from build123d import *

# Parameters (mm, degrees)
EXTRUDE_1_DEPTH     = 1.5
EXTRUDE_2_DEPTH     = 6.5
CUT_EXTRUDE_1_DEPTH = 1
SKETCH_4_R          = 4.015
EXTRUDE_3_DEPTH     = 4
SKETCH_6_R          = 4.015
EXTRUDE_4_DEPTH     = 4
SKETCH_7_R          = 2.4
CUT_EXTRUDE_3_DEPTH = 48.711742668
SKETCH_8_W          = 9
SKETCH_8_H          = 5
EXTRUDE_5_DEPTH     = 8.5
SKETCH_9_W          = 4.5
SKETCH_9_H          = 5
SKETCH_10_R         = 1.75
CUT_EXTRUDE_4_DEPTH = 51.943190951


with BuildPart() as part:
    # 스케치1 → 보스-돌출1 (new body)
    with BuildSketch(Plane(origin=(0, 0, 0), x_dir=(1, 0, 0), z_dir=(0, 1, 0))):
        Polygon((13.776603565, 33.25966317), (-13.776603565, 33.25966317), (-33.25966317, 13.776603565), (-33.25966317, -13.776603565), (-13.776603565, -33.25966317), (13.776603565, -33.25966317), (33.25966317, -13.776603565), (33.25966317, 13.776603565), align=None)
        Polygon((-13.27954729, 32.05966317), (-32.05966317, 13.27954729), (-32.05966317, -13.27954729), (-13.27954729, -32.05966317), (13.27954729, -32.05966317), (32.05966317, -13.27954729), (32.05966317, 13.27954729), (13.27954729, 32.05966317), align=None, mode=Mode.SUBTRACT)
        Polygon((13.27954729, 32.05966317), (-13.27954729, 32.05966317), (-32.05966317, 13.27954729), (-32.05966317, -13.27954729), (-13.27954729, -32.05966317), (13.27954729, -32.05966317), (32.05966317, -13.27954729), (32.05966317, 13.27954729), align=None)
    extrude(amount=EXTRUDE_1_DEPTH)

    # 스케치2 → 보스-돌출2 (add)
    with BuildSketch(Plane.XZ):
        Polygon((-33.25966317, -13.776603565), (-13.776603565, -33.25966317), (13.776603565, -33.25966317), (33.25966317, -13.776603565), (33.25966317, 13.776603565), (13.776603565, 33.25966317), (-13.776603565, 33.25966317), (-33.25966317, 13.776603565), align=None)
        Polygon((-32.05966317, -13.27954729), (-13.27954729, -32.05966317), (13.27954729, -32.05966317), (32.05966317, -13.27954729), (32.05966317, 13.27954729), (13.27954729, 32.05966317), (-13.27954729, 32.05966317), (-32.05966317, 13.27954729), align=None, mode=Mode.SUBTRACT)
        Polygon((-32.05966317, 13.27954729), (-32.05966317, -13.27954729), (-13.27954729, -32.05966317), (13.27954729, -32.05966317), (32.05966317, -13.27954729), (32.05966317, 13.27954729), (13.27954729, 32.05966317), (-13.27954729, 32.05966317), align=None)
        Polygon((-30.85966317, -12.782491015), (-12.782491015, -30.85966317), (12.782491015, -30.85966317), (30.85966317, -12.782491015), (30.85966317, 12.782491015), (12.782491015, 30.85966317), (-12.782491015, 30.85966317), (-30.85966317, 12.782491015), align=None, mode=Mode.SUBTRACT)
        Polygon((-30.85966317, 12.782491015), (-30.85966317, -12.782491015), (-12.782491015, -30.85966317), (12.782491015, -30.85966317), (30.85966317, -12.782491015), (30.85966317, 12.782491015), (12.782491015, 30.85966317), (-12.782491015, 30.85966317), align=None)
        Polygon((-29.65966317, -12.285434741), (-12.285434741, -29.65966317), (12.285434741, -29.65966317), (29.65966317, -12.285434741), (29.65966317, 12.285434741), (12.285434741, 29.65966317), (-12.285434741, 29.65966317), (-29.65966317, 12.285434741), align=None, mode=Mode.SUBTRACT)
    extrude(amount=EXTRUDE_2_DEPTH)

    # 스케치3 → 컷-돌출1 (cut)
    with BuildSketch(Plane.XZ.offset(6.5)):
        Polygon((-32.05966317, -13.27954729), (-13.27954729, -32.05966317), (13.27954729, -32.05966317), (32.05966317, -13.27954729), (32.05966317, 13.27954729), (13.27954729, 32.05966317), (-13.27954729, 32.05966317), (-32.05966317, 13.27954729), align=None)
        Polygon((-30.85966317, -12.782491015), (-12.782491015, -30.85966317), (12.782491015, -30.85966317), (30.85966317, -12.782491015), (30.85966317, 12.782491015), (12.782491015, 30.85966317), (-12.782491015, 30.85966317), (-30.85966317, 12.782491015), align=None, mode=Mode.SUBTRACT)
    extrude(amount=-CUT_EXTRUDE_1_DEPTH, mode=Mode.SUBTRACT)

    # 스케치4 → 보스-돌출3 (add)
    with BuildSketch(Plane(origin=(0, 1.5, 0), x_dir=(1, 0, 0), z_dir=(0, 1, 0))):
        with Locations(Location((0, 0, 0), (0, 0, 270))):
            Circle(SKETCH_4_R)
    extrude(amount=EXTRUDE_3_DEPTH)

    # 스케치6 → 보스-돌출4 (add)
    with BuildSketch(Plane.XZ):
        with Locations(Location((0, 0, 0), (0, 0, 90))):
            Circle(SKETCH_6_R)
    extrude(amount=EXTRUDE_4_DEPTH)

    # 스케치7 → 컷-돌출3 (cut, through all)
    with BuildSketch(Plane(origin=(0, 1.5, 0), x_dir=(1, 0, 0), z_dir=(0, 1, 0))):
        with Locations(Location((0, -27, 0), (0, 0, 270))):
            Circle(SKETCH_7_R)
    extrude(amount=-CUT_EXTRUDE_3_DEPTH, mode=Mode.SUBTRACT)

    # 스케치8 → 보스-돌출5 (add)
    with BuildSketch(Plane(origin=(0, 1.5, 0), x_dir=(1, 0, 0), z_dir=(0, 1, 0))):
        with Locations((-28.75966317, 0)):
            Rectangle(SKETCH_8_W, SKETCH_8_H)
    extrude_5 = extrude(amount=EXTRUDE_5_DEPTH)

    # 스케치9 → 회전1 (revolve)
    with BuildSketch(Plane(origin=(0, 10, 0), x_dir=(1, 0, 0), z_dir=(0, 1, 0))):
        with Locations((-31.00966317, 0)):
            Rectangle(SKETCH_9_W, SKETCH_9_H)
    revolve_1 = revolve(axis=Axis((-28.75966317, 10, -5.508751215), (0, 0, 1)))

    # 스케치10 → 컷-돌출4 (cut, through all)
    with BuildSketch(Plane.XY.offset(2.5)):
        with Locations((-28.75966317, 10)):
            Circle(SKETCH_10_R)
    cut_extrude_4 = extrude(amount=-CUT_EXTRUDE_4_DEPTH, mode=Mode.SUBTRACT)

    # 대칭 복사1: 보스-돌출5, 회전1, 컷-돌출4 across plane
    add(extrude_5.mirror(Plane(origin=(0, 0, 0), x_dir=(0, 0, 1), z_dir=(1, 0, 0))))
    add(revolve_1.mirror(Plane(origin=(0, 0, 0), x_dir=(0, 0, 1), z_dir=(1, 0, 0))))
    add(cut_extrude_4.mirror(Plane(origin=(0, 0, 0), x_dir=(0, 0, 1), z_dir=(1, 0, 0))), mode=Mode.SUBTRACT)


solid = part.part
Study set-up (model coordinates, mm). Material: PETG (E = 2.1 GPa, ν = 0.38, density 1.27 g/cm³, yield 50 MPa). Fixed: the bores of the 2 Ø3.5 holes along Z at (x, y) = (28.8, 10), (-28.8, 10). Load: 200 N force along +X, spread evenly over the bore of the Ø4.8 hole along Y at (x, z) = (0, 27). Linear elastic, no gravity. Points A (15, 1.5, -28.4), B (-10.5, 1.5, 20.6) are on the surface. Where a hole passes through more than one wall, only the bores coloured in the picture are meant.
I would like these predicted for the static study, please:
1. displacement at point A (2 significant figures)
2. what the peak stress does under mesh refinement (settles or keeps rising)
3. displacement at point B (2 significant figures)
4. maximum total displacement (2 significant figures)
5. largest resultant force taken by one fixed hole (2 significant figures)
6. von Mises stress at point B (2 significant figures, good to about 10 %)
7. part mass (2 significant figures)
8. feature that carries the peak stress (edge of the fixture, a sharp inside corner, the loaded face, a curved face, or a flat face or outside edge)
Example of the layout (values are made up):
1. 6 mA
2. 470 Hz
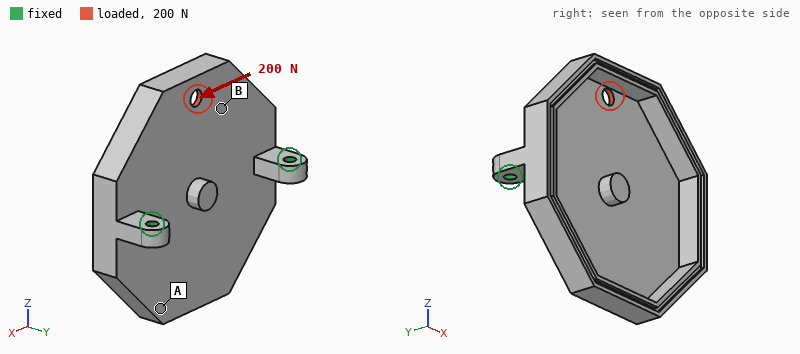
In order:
1. 0.13 mm
2. keeps rising
3. 0.26 mm
4. 0.35 mm
5. 140 N
6. 5.3 MPa
7. 15 g
8. edge of the fixture
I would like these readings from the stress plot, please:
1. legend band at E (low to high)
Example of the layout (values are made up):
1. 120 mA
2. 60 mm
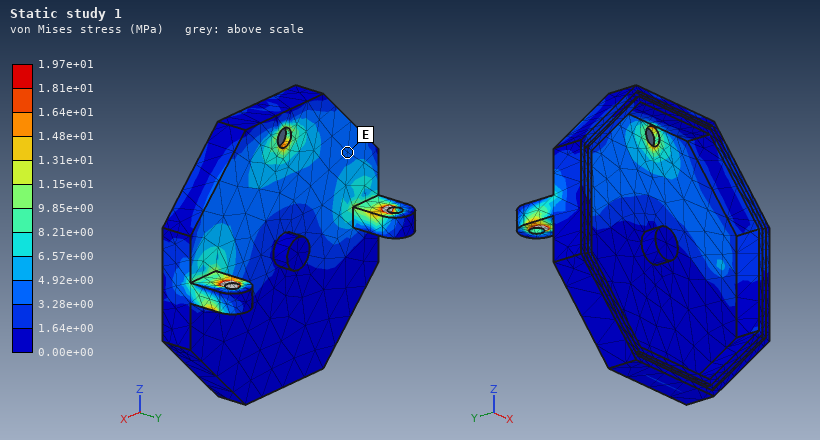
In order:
1. 3.28e+00 to 4.92e+00 MPa
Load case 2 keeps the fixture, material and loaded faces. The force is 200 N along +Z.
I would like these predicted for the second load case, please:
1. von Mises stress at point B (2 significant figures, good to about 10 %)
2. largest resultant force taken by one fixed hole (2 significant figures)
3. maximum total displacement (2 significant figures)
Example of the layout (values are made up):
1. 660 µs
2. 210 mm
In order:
1. 3.8 MPa
2. 100 N
3. 0.67 mm
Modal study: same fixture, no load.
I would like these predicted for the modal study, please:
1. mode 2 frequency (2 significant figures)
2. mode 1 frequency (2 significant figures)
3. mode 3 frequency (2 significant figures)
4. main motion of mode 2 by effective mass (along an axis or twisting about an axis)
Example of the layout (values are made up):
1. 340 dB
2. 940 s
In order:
1. 640 Hz
2. 350 Hz
3. 1000 Hz
4. along Y
